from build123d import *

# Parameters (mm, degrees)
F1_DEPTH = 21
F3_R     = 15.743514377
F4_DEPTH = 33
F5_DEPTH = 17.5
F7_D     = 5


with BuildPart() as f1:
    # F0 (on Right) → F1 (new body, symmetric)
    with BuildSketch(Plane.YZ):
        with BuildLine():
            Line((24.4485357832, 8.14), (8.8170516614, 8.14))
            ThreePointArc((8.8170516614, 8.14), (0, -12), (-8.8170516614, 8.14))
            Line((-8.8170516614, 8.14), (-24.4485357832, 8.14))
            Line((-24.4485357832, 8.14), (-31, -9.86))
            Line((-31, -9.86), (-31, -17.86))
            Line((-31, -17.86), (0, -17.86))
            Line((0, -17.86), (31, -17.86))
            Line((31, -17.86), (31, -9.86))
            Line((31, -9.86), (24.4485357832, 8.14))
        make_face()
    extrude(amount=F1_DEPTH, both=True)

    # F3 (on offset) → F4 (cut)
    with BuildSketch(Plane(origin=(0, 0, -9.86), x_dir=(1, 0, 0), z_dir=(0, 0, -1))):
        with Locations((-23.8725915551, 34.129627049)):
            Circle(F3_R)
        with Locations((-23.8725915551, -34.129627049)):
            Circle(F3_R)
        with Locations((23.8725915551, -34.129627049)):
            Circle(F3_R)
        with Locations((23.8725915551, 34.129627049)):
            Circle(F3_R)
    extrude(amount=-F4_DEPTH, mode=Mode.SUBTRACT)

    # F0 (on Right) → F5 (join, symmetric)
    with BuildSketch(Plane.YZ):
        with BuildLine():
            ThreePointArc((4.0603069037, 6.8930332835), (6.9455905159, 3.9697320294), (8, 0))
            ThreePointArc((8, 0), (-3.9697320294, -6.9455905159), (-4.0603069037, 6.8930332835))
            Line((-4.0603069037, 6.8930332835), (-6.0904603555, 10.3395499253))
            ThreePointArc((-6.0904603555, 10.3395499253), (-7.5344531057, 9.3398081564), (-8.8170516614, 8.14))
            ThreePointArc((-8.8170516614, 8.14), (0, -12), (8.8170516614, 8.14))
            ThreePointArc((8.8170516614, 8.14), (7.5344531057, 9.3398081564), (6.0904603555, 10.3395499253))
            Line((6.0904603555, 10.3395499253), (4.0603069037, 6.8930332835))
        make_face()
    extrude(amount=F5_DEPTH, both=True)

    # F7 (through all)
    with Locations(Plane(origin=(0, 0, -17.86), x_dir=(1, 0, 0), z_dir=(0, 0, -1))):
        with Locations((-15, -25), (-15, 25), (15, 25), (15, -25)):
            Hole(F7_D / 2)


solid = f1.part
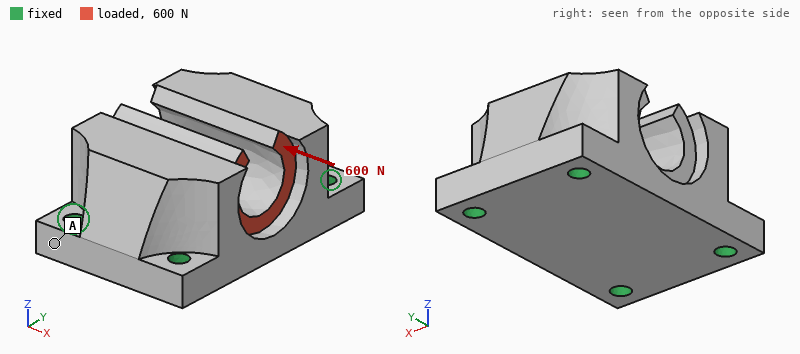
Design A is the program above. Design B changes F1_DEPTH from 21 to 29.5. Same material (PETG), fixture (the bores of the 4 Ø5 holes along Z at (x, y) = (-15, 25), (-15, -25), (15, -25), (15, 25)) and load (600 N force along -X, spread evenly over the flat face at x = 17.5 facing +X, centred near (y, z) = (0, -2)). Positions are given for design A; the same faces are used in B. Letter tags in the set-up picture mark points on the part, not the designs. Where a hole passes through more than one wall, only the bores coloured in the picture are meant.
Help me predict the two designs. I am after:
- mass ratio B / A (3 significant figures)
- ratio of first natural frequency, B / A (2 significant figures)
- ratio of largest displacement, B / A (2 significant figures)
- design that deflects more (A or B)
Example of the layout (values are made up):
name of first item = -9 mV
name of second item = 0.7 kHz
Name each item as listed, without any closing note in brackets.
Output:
mass ratio B / A = 1.27
ratio of first natural frequency, B / A = 0.95
ratio of largest displacement, B / A = 0.89
design that deflects more = A
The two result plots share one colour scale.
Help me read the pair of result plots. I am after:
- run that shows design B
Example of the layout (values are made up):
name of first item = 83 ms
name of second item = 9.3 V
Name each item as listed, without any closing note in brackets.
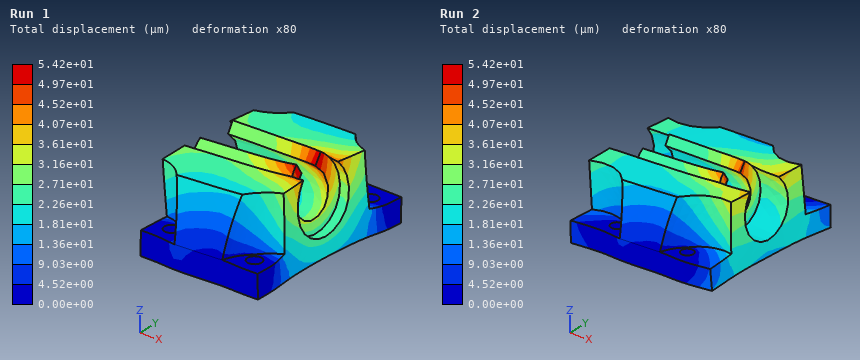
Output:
run that shows design B = Run 2
